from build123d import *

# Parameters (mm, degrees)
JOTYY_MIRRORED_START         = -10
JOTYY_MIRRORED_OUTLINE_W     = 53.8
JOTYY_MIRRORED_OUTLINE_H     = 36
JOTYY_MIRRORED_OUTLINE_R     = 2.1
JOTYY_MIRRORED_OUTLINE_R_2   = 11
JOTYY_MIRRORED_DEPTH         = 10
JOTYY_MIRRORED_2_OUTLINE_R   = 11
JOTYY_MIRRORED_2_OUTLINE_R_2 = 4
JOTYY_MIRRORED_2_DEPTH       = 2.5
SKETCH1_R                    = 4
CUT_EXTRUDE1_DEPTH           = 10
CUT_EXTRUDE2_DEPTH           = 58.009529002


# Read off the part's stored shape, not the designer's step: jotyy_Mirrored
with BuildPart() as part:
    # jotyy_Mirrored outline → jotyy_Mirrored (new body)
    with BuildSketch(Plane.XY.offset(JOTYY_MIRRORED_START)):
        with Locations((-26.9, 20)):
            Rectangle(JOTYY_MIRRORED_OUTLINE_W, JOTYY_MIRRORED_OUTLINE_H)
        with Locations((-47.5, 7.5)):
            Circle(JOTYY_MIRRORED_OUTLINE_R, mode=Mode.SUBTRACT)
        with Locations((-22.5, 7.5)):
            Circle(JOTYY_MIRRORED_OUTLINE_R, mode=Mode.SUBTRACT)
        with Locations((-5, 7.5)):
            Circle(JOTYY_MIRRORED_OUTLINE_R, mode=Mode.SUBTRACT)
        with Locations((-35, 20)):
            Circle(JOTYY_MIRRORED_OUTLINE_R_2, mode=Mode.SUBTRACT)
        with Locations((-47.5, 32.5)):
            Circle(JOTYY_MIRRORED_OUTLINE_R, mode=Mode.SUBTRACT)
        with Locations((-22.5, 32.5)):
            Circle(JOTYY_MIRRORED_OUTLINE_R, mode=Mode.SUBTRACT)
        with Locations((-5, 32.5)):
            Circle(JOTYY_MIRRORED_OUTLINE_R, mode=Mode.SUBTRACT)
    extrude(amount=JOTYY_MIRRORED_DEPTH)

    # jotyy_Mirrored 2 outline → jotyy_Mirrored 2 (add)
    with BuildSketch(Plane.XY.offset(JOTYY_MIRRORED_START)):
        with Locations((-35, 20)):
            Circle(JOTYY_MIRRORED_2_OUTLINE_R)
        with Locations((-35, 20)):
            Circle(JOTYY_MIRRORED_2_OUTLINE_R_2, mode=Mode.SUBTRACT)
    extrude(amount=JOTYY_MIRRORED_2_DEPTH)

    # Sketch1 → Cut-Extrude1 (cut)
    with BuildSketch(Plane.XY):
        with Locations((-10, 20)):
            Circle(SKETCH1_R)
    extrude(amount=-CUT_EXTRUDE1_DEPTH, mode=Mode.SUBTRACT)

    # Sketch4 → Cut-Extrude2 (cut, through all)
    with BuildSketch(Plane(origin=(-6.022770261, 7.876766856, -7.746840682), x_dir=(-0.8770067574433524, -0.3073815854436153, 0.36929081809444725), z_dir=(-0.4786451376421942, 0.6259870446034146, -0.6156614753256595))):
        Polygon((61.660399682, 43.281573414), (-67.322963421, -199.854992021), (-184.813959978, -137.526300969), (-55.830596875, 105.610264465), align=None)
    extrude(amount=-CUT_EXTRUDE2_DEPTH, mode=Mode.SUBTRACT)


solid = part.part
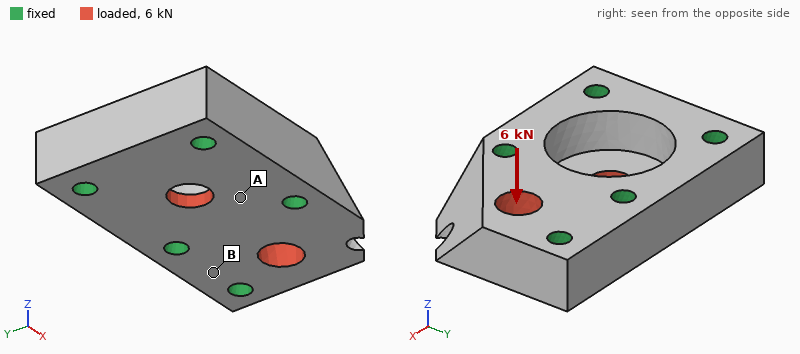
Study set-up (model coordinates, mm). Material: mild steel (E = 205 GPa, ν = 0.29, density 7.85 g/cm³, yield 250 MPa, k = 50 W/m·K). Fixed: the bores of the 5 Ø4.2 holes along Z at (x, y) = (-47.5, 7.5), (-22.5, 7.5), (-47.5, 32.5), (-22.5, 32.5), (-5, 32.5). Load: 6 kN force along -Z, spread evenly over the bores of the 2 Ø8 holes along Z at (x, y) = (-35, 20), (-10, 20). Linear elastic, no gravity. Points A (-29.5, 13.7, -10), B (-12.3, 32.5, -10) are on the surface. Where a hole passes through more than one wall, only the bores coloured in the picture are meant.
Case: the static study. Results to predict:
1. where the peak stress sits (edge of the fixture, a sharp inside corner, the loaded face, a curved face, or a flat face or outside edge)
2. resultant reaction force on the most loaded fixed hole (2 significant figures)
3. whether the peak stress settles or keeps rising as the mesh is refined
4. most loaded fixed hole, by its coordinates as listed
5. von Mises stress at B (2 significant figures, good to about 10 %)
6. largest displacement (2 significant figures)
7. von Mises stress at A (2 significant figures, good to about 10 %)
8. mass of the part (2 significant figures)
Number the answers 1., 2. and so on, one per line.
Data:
1. edge of the fixture
2. 2.4 kN
3. keeps rising
4. (-5, 32.5)
5. 20 MPa
6. 12 µm
7. 65 MPa
8. 110 g
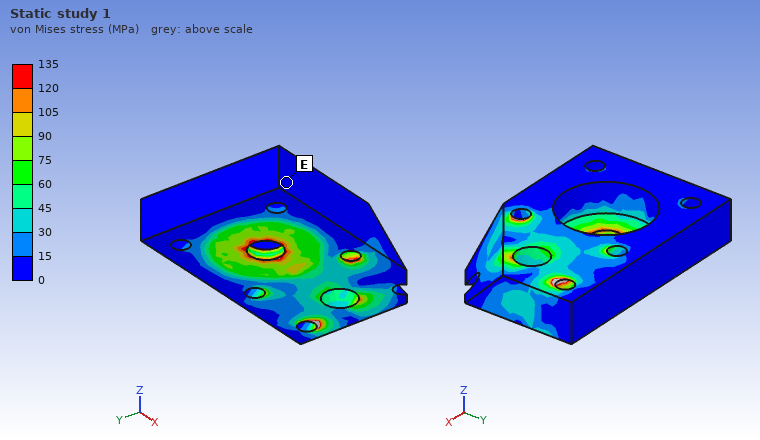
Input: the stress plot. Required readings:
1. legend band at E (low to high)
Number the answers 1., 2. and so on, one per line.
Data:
1. 0 to 15 MPa
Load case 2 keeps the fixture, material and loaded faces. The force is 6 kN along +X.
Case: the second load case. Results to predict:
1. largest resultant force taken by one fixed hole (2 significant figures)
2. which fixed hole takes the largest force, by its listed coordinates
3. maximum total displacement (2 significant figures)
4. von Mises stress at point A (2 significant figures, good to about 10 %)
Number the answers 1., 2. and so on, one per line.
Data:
1. 2.3 kN
2. (-22.5, 7.5)
3. 2.8 µm
4. 17 MPa
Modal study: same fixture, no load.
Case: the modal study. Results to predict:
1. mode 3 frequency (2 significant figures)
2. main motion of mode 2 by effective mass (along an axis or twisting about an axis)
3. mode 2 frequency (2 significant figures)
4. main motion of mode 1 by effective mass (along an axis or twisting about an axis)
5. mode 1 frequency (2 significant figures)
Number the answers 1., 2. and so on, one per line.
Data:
1. 50 kHz
2. along Z
3. 40 kHz
4. along Z
5. 29 kHz
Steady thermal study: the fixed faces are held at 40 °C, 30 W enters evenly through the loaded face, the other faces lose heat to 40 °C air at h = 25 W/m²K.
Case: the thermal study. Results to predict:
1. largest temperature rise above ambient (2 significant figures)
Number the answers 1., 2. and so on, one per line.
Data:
1. 22 K
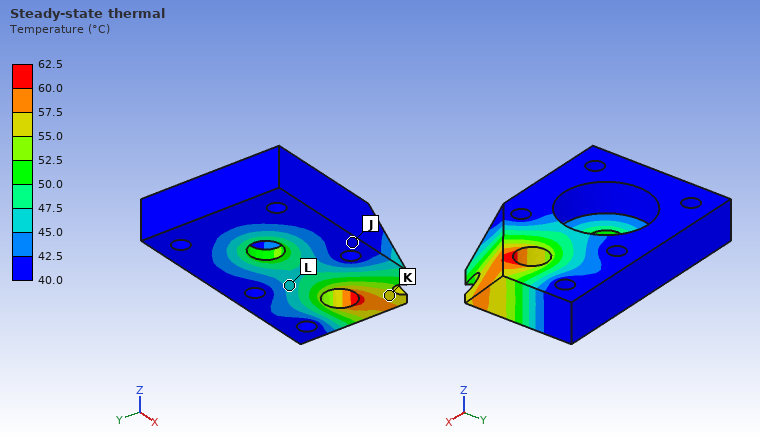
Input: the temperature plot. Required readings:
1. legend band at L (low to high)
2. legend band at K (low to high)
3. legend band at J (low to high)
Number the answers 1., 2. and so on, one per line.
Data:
1. 45.0 to 47.5 °C
2. 55.0 to 57.5 °C
3. 40.0 to 42.5 °C
